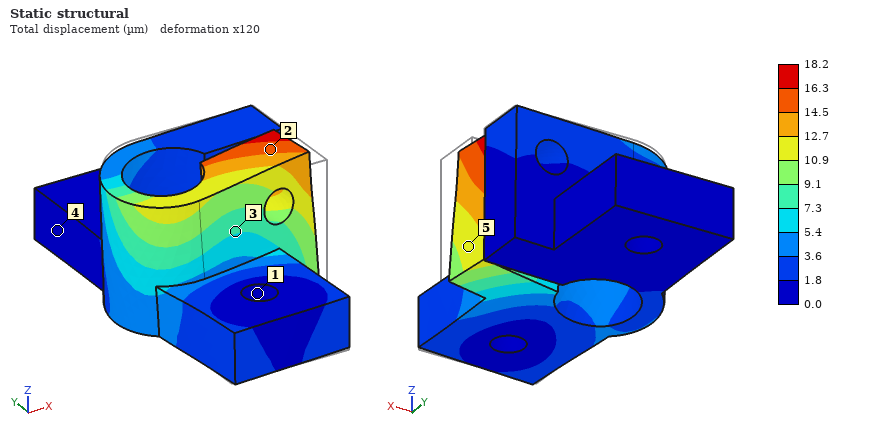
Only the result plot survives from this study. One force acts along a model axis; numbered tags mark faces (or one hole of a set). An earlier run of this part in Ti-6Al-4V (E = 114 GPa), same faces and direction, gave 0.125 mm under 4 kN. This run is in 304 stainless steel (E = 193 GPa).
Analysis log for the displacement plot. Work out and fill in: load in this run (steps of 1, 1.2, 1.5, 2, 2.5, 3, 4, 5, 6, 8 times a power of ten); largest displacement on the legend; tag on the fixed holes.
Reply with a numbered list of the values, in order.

1. 1 kN
2. 18.2 µm
3. 1
